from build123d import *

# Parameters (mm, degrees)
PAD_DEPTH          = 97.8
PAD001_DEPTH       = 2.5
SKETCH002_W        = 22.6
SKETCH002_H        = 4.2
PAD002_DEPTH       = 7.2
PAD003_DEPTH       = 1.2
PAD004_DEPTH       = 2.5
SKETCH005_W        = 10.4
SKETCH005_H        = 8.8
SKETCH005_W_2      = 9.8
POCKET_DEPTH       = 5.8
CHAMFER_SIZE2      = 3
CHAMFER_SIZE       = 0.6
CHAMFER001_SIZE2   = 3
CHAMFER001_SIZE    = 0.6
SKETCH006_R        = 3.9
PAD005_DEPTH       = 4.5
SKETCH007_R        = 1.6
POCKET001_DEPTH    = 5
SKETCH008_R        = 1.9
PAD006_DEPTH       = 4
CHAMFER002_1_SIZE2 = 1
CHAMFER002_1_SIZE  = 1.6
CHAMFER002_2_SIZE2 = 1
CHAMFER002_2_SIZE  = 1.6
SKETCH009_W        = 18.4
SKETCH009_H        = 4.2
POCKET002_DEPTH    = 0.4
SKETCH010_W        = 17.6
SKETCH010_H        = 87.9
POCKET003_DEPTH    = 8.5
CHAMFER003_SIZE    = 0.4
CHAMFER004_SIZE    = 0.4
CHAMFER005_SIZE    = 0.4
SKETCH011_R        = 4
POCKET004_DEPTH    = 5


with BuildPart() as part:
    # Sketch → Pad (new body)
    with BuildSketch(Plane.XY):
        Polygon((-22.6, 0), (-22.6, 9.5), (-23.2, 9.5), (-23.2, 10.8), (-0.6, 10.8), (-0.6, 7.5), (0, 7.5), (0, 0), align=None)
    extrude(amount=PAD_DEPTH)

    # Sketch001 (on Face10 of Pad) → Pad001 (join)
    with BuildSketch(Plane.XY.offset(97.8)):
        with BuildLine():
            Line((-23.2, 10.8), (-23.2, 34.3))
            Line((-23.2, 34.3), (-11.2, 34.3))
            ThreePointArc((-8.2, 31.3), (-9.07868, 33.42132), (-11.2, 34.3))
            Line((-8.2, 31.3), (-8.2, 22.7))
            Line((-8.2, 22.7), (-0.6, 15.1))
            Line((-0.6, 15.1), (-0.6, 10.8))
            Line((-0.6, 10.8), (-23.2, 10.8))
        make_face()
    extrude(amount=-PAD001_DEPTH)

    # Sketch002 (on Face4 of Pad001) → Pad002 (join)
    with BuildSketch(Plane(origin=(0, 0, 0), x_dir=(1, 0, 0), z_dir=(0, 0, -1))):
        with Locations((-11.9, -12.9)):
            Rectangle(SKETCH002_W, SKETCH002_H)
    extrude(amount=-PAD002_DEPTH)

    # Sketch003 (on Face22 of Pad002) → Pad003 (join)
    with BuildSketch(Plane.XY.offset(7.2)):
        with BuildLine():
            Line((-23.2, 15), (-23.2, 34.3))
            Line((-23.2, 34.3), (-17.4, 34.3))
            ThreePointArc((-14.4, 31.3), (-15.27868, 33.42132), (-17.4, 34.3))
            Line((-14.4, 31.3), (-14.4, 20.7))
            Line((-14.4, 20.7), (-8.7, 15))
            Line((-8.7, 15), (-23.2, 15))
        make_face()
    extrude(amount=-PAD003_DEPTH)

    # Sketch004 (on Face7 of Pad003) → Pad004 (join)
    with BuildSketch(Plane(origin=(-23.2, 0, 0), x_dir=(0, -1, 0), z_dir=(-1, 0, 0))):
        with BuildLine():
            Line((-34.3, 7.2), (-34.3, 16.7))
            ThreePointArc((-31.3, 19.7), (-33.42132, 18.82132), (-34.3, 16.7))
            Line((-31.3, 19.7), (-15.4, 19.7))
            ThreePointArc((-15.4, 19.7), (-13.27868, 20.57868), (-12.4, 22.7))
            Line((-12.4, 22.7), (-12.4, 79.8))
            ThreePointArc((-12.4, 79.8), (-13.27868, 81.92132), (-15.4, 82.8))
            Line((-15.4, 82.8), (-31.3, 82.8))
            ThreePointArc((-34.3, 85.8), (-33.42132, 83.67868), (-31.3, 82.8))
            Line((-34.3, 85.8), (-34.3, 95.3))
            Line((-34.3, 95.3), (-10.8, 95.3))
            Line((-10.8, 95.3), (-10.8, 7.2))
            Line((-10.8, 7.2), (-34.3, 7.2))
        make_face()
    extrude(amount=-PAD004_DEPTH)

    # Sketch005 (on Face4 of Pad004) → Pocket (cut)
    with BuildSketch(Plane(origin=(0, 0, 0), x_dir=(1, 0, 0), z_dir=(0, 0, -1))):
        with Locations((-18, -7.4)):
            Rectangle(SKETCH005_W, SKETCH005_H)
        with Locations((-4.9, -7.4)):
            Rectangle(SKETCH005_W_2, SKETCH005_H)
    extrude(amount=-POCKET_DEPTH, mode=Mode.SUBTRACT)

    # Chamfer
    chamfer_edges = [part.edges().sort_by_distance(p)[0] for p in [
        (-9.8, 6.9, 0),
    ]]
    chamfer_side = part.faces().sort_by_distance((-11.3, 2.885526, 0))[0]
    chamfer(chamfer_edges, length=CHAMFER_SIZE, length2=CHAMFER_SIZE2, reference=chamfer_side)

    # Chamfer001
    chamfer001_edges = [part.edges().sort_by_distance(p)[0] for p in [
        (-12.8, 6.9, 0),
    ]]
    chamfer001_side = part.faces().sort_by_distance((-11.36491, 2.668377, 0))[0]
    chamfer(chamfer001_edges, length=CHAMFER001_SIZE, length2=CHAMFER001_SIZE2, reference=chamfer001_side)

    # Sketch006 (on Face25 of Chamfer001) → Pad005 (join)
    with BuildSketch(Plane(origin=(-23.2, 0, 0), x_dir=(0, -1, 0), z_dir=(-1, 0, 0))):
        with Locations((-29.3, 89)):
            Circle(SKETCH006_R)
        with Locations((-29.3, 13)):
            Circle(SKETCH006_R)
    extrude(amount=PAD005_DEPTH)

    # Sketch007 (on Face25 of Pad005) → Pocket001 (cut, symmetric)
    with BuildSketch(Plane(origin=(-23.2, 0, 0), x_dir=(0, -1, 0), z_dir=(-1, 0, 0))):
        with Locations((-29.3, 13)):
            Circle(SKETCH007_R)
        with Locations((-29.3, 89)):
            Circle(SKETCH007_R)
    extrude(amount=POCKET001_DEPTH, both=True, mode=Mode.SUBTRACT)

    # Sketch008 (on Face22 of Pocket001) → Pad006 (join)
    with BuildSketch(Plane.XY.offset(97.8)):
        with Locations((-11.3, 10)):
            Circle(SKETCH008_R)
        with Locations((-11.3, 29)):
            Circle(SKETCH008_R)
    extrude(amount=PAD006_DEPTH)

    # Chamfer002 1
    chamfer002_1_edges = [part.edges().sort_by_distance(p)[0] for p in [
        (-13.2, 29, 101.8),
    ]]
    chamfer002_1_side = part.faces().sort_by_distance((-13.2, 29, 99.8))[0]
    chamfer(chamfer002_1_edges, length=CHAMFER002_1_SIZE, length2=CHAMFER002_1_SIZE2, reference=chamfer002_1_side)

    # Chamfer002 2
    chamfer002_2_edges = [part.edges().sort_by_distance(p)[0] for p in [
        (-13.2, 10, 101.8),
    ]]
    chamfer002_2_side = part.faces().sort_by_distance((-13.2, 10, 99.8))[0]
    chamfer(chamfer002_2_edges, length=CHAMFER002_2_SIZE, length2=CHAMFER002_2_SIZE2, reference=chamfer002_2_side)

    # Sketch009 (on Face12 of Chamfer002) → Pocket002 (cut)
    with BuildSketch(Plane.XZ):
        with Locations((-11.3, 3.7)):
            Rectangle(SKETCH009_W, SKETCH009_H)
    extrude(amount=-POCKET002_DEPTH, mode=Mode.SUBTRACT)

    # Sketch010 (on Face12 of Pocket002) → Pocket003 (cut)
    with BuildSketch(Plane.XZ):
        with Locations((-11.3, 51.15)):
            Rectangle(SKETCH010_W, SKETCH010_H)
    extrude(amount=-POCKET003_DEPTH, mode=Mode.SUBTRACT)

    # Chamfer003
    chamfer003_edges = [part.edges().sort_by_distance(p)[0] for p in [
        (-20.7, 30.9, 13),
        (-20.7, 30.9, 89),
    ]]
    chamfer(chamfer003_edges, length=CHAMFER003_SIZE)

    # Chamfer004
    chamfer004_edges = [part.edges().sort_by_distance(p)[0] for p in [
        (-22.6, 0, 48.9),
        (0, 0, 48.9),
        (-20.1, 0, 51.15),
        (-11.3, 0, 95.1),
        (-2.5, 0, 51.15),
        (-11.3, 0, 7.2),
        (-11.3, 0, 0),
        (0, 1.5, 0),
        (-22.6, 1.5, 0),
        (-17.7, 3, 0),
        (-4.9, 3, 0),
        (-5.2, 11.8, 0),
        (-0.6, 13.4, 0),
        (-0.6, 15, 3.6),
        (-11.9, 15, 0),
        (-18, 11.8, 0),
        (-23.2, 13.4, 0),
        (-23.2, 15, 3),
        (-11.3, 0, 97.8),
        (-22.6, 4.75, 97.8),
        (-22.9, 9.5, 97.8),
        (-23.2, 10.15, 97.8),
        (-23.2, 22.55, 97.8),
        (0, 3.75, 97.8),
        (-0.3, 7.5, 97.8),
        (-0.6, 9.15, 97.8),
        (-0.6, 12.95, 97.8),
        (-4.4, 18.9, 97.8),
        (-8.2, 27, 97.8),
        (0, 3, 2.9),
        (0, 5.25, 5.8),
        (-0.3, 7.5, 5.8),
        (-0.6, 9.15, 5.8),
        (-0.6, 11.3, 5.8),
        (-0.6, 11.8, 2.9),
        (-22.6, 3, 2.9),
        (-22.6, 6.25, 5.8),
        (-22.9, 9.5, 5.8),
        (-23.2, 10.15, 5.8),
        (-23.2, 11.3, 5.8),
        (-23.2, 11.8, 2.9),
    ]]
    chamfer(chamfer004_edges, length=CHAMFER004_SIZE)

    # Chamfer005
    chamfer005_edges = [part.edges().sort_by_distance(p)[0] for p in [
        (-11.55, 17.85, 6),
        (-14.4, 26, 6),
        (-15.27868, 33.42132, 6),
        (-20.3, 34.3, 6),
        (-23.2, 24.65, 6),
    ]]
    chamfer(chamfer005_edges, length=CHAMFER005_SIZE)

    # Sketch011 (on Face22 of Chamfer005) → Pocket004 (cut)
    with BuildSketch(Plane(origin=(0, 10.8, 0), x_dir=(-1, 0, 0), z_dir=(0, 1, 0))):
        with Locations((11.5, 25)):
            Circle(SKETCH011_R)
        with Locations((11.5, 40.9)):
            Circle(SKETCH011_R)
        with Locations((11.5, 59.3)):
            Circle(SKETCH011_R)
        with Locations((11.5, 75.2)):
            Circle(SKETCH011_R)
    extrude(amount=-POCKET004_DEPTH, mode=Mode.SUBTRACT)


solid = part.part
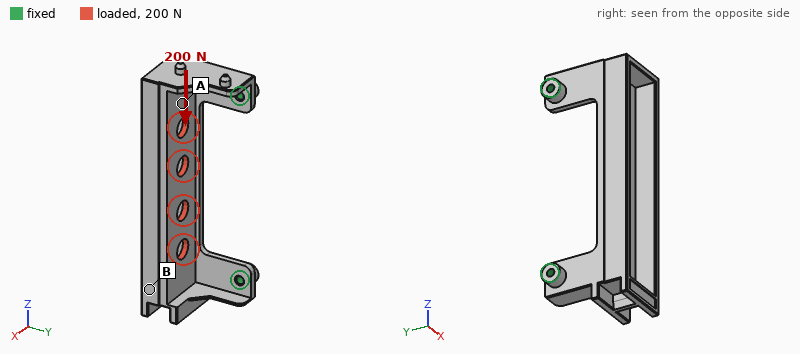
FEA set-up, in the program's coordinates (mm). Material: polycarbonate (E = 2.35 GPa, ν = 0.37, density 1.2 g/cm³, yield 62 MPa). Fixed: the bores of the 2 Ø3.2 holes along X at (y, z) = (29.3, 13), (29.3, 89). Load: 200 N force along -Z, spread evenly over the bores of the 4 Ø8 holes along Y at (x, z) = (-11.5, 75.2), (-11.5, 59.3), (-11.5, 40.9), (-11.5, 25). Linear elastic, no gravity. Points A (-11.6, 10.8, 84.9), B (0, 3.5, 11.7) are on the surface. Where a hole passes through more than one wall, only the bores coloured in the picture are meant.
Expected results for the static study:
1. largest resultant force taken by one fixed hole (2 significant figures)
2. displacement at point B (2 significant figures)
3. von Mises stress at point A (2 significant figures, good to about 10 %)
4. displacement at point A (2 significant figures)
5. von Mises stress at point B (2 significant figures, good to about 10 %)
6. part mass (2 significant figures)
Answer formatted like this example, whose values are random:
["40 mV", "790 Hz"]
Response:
["110 N", "0.72 mm", "3.9 MPa", "0.46 mm", "2.1 MPa", "16 g"]
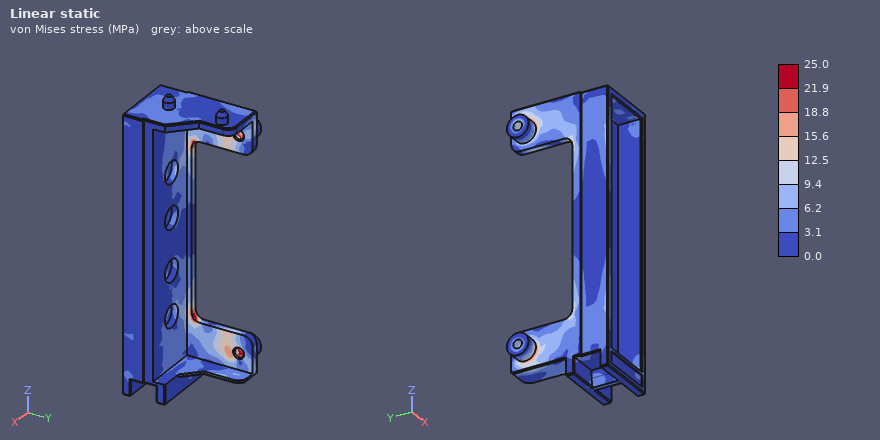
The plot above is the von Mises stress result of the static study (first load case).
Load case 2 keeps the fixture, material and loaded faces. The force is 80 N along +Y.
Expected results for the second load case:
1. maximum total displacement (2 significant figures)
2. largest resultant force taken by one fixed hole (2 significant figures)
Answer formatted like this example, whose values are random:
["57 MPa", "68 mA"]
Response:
["1.2 mm", "43 N"]
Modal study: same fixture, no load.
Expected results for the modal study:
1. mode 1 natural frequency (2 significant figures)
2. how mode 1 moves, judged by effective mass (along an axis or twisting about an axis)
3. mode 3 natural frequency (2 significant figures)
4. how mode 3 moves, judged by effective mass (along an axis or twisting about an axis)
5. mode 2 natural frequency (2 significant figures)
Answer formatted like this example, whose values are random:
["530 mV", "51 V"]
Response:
["330 Hz", "along X", "1100 Hz", "along Z", "500 Hz"]
